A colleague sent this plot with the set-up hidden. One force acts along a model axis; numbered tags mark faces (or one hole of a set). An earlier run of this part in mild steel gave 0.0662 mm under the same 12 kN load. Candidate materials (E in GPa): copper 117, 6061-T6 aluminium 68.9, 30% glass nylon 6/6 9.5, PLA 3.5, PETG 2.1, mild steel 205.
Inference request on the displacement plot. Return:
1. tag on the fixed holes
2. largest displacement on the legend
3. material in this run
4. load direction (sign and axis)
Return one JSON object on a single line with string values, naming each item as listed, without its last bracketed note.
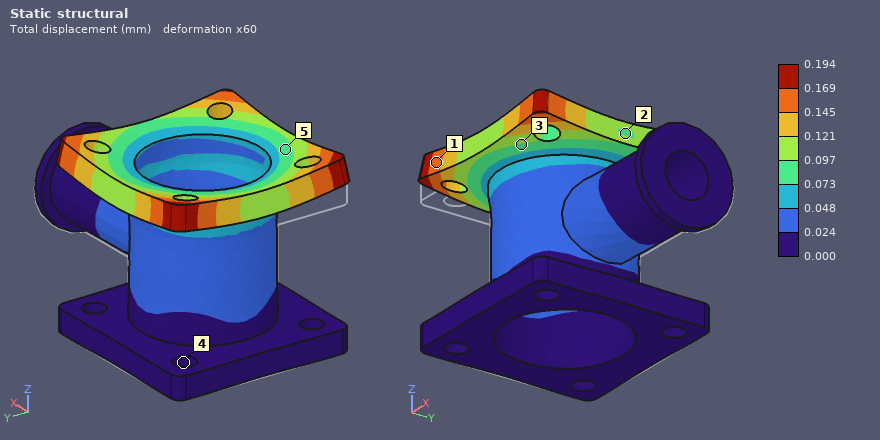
{"tag on the fixed holes": "4", "largest displacement on the legend": "0.194 mm", "material in this run": "6061-T6 aluminium", "load direction": "+Z"}
